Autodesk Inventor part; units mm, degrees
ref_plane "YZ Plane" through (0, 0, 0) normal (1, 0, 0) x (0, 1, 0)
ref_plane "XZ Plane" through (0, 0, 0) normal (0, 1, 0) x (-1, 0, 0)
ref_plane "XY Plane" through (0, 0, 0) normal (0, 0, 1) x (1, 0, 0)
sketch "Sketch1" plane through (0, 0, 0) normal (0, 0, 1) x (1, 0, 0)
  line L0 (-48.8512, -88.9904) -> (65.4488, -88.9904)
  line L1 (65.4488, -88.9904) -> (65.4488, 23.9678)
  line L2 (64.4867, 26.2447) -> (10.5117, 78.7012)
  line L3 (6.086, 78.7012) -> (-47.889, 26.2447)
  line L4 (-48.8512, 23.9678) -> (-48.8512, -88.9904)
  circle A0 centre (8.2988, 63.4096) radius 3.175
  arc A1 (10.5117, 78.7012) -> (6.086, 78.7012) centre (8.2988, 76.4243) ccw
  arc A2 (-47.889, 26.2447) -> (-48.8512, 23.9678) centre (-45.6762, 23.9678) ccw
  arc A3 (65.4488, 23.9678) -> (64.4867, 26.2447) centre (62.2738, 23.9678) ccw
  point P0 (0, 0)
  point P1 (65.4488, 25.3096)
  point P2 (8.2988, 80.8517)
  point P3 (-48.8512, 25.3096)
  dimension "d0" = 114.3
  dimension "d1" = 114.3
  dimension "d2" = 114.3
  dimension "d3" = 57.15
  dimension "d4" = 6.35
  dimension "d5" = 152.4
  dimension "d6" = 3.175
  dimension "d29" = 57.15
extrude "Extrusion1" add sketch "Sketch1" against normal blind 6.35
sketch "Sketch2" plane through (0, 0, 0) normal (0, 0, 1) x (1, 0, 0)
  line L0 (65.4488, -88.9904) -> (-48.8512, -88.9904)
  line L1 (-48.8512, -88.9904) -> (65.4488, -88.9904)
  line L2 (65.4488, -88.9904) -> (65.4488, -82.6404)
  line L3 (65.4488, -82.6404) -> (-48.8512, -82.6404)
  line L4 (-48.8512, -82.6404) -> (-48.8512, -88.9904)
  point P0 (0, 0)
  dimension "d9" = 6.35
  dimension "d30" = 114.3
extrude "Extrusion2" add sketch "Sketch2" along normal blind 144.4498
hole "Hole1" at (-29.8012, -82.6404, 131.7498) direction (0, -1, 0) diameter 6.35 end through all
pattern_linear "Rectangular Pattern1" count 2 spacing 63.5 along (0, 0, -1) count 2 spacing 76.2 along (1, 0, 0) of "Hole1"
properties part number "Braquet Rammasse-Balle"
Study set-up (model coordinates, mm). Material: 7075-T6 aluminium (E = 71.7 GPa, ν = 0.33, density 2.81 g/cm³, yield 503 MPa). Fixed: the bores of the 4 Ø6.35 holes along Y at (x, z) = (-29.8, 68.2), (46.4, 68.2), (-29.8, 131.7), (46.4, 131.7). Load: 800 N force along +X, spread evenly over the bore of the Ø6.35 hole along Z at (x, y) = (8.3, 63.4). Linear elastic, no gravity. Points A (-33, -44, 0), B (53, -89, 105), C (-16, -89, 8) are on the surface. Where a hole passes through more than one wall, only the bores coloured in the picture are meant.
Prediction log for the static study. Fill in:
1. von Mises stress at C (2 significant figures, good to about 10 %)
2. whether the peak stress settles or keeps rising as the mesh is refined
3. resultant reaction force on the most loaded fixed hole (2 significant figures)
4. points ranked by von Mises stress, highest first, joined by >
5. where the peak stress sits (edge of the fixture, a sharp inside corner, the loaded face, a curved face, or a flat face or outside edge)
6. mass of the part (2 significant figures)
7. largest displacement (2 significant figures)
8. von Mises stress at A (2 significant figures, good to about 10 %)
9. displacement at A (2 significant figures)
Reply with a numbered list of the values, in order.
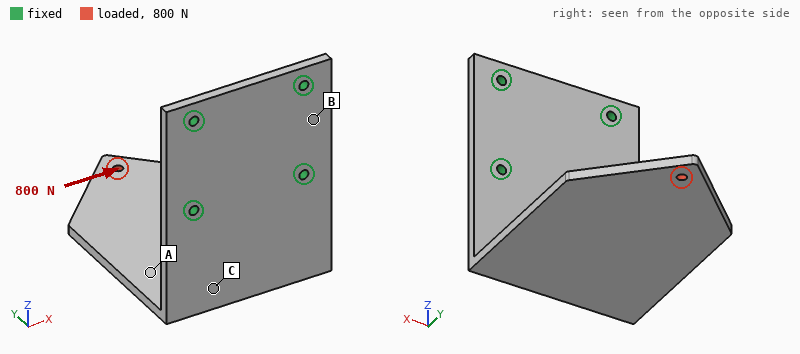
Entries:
1. 76 MPa
2. keeps rising
3. 1.7 kN
4. C > A > B
5. edge of the fixture
6. 580 g
7. 2.7 mm
8. 25 MPa
9. 0.98 mm
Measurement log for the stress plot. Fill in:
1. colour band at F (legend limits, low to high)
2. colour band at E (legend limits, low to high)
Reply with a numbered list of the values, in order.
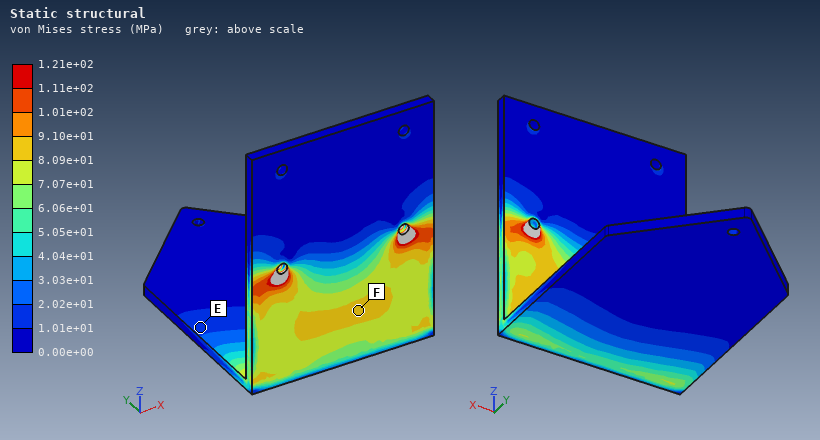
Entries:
1. 8.09e+01 to 9.10e+01 MPa
2. 1.01e+01 to 2.02e+01 MPa
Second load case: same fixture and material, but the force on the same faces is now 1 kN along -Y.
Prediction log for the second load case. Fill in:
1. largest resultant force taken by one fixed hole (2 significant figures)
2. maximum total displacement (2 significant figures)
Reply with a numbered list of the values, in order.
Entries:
1. 680 N
2. 2.6 mm
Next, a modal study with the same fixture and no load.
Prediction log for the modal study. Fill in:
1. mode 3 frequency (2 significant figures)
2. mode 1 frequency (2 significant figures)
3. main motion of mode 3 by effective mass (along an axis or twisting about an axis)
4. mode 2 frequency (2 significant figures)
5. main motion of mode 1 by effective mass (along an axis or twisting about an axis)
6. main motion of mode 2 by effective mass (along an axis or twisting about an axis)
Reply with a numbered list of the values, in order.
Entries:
1. 480 Hz
2. 140 Hz
3. along Y
4. 290 Hz
5. along Z
6. along X
